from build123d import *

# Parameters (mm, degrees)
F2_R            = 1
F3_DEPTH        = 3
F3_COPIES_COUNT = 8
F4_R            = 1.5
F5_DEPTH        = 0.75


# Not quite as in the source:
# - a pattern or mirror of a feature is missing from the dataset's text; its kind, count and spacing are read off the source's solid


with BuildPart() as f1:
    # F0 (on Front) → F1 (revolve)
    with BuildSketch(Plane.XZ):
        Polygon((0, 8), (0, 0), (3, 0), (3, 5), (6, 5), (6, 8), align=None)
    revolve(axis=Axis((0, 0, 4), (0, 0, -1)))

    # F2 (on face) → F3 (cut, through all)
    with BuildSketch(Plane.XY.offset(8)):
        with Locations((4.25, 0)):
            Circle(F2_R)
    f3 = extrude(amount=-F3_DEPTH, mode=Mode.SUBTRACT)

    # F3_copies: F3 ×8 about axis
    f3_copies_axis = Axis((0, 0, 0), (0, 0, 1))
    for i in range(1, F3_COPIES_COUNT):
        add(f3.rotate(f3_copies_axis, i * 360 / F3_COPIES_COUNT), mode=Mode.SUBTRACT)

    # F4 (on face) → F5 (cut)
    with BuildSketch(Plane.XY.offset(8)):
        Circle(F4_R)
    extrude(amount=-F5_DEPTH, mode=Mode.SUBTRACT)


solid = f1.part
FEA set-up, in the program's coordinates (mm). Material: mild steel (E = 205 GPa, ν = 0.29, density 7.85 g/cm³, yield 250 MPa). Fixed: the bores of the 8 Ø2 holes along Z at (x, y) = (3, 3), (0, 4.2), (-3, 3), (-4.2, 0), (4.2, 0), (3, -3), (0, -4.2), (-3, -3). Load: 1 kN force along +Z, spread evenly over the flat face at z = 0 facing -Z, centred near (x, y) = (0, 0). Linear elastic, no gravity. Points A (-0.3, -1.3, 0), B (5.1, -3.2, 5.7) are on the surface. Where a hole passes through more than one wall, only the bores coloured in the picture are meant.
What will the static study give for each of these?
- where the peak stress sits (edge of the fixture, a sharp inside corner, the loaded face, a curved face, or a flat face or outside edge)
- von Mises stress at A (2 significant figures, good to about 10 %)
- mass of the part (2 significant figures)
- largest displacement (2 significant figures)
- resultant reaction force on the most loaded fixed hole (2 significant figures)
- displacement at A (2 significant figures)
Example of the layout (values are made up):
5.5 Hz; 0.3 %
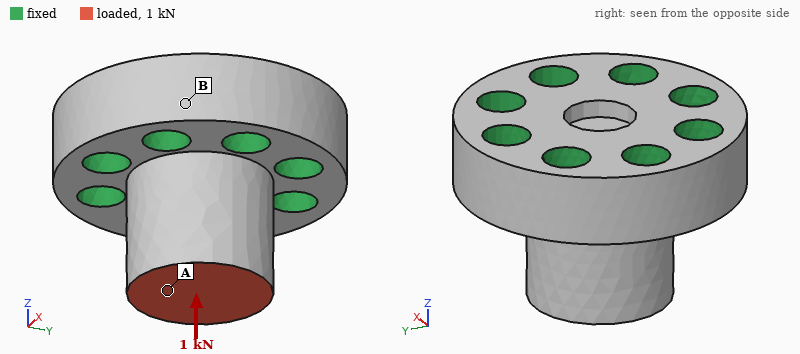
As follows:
edge of the fixture; 36 MPa; 3.1 g; 1.2 µm; 140 N; 1.2 µm
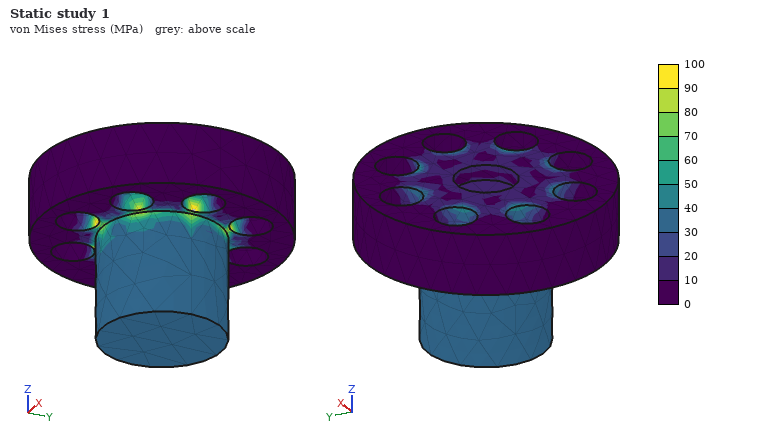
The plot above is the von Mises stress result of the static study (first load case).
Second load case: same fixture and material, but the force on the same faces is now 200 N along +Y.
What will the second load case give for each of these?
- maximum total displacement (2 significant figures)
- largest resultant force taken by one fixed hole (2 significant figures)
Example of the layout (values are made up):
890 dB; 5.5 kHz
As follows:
1.8 µm; 100 N
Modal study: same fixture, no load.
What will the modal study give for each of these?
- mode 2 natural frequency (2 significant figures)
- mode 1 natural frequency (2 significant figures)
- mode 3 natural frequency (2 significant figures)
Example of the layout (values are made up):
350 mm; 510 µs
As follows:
89 kHz; 89 kHz; 140 kHz
